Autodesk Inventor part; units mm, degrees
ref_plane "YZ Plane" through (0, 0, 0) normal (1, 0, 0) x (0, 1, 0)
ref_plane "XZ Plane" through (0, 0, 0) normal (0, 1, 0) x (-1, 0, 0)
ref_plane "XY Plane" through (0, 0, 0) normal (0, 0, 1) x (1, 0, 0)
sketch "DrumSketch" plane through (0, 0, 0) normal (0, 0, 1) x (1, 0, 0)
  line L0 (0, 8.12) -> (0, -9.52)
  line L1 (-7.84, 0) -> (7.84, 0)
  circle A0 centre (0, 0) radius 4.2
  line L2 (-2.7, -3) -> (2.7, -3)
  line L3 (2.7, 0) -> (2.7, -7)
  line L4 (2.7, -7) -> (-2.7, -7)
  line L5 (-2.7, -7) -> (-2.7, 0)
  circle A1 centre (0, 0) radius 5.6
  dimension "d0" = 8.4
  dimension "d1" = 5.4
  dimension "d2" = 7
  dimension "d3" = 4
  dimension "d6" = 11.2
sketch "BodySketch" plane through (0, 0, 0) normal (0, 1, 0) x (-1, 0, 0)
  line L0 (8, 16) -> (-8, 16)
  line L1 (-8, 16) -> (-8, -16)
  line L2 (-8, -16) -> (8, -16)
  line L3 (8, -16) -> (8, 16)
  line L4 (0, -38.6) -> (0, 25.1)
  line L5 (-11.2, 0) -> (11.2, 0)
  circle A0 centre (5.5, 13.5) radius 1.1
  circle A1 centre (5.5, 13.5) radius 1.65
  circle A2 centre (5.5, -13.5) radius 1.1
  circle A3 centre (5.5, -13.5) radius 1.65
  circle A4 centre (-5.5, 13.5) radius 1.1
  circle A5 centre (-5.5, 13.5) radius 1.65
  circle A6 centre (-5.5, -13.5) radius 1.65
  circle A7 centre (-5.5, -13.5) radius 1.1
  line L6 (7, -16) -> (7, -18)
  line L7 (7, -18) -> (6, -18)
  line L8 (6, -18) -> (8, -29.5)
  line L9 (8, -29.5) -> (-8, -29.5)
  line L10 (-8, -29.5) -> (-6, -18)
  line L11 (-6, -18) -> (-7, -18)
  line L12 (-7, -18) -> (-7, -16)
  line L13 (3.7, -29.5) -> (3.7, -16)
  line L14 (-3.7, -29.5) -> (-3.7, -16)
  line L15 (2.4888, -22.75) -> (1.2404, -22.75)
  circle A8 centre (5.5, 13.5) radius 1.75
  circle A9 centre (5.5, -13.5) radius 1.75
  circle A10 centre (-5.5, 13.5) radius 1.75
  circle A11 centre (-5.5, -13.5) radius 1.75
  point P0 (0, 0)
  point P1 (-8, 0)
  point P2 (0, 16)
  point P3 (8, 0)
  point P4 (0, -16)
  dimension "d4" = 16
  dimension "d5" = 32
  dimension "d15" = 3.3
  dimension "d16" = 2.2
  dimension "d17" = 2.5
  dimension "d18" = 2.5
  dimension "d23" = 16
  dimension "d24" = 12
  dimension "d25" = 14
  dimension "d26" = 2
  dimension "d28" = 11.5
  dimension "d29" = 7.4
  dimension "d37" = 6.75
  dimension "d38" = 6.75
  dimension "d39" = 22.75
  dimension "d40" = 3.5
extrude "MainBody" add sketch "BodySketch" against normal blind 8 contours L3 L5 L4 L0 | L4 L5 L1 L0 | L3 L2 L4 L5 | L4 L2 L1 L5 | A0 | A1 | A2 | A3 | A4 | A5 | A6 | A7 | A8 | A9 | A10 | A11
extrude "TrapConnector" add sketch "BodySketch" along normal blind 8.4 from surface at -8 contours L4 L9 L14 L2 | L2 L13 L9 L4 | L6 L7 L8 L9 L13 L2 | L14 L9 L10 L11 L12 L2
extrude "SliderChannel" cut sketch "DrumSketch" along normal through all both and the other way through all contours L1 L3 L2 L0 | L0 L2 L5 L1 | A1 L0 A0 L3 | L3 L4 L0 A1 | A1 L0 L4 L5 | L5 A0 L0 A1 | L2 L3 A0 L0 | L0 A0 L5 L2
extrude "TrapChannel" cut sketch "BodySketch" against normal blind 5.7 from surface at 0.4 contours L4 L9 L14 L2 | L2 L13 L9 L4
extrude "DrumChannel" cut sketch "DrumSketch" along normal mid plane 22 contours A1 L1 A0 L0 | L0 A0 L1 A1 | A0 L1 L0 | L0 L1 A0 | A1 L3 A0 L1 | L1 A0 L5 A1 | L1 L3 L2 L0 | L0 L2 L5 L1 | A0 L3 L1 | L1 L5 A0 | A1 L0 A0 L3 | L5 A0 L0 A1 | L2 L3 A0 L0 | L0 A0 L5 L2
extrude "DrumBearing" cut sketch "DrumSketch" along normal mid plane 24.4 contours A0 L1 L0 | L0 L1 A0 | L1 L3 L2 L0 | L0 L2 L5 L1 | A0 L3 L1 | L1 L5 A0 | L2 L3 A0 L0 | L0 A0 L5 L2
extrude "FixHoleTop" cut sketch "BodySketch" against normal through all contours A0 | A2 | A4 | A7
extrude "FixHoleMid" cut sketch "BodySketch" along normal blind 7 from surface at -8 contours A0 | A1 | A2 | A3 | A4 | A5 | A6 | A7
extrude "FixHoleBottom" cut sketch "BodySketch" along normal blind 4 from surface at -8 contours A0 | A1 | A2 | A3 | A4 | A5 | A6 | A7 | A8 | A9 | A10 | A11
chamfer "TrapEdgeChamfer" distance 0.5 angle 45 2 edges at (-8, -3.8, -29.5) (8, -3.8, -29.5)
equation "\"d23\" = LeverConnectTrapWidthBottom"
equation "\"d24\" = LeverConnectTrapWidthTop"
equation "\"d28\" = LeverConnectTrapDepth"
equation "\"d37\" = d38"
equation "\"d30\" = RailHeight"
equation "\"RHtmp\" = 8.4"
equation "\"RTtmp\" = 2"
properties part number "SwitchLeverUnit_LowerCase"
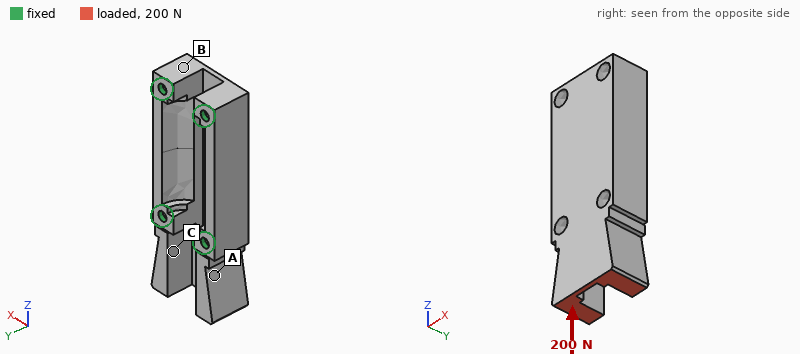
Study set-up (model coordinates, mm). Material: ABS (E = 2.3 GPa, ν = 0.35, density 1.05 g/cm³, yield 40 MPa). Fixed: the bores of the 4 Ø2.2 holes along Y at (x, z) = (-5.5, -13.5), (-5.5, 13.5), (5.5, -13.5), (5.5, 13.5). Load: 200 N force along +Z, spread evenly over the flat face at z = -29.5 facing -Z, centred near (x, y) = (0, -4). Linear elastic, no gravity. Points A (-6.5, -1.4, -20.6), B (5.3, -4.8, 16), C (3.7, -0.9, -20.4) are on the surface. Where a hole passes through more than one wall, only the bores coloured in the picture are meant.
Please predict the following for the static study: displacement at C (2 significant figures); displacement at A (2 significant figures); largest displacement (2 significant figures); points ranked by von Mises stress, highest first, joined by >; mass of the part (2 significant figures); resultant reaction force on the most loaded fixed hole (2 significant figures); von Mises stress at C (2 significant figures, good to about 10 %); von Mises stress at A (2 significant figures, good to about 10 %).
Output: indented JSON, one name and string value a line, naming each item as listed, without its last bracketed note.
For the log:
{
  "displacement at C": "0.039 mm",
  "displacement at A": "0.043 mm",
  "largest displacement": "0.11 mm",
  "points ranked by von Mises stress, highest first, joined by >": "A > C > B",
  "mass of the part": "3.2 g",
  "resultant reaction force on the most loaded fixed hole": "68 N",
  "von Mises stress at C": "2.9 MPa",
  "von Mises stress at A": "4.6 MPa"
}
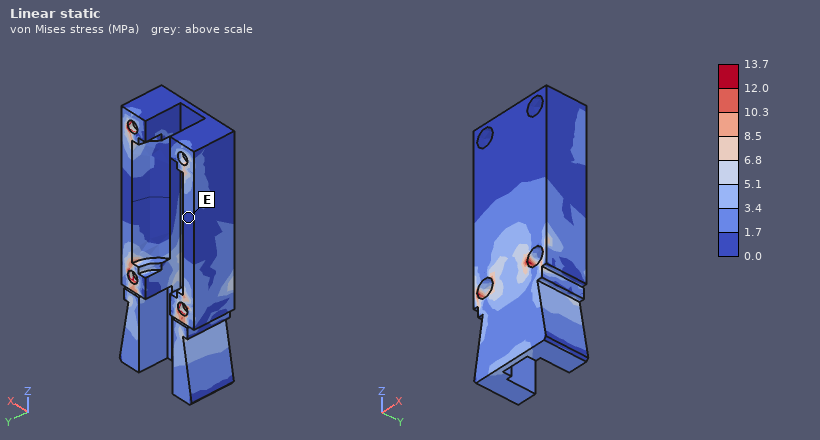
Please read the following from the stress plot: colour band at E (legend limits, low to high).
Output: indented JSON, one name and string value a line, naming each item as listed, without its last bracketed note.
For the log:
{
  "colour band at E": "0.0 to 1.7 MPa"
}
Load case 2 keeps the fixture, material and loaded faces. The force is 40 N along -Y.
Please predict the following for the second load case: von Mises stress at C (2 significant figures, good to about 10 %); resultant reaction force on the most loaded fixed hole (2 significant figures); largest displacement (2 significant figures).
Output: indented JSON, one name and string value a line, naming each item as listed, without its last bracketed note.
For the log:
{
  "von Mises stress at C": "3.1 MPa",
  "resultant reaction force on the most loaded fixed hole": "39 N",
  "largest displacement": "0.17 mm"
}
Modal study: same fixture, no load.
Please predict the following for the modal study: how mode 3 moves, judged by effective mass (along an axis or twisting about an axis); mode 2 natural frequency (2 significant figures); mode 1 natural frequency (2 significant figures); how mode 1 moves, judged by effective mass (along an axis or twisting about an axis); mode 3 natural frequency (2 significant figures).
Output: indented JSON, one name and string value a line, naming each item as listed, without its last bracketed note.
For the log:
{
  "how mode 3 moves, judged by effective mass": "along X",
  "mode 2 natural frequency": "3900 Hz",
  "mode 1 natural frequency": "3300 Hz",
  "how mode 1 moves, judged by effective mass": "along X",
  "mode 3 natural frequency": "4200 Hz"
}
